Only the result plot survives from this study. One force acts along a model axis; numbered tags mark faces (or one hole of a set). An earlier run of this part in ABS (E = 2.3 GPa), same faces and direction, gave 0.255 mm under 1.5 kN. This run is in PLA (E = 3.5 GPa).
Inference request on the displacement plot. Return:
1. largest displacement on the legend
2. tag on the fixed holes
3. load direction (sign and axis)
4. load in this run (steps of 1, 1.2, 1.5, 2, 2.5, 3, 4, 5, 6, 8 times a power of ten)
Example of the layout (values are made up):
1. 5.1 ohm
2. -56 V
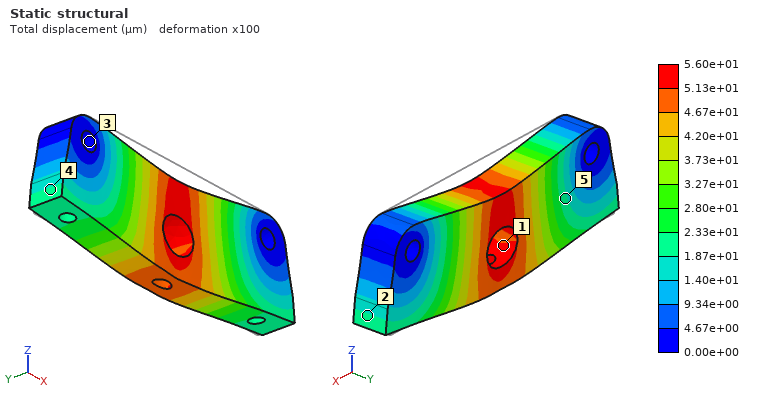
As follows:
1. 5.60e+01 µm
2. 3
3. -Z
4. 500 N
